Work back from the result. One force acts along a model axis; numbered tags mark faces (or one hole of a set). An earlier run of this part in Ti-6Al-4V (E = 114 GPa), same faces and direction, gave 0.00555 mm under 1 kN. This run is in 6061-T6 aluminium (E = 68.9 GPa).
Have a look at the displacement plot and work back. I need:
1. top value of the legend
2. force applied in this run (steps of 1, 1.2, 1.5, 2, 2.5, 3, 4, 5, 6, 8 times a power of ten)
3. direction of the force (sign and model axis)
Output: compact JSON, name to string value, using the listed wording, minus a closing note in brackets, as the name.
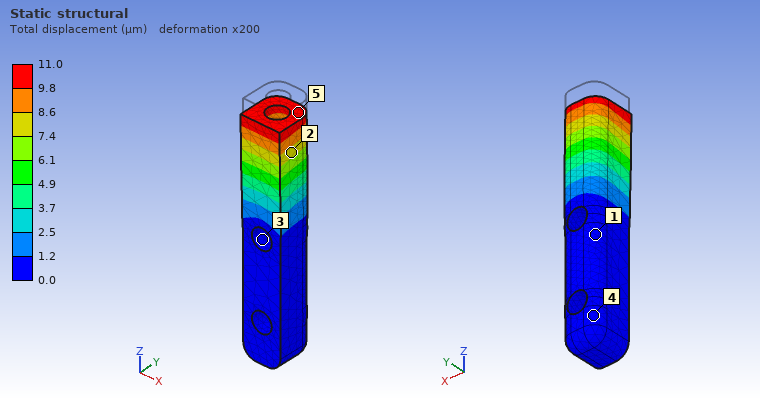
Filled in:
{"top value of the legend": "11.0 µm", "force applied in this run": "1.2 kN", "direction of the force": "-Z"}
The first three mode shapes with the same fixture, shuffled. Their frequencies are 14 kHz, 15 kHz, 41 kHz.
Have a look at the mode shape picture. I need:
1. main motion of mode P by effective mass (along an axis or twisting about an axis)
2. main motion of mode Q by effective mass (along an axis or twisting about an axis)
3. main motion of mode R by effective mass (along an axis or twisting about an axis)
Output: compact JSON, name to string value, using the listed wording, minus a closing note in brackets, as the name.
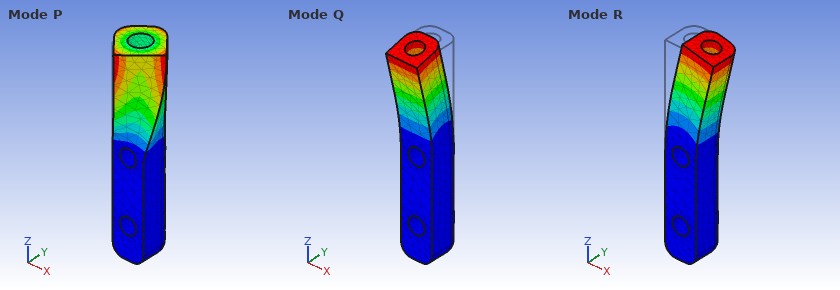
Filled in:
{"main motion of mode P by effective mass": "twisting about Z", "main motion of mode Q by effective mass": "along Y", "main motion of mode R by effective mass": "along X"}
